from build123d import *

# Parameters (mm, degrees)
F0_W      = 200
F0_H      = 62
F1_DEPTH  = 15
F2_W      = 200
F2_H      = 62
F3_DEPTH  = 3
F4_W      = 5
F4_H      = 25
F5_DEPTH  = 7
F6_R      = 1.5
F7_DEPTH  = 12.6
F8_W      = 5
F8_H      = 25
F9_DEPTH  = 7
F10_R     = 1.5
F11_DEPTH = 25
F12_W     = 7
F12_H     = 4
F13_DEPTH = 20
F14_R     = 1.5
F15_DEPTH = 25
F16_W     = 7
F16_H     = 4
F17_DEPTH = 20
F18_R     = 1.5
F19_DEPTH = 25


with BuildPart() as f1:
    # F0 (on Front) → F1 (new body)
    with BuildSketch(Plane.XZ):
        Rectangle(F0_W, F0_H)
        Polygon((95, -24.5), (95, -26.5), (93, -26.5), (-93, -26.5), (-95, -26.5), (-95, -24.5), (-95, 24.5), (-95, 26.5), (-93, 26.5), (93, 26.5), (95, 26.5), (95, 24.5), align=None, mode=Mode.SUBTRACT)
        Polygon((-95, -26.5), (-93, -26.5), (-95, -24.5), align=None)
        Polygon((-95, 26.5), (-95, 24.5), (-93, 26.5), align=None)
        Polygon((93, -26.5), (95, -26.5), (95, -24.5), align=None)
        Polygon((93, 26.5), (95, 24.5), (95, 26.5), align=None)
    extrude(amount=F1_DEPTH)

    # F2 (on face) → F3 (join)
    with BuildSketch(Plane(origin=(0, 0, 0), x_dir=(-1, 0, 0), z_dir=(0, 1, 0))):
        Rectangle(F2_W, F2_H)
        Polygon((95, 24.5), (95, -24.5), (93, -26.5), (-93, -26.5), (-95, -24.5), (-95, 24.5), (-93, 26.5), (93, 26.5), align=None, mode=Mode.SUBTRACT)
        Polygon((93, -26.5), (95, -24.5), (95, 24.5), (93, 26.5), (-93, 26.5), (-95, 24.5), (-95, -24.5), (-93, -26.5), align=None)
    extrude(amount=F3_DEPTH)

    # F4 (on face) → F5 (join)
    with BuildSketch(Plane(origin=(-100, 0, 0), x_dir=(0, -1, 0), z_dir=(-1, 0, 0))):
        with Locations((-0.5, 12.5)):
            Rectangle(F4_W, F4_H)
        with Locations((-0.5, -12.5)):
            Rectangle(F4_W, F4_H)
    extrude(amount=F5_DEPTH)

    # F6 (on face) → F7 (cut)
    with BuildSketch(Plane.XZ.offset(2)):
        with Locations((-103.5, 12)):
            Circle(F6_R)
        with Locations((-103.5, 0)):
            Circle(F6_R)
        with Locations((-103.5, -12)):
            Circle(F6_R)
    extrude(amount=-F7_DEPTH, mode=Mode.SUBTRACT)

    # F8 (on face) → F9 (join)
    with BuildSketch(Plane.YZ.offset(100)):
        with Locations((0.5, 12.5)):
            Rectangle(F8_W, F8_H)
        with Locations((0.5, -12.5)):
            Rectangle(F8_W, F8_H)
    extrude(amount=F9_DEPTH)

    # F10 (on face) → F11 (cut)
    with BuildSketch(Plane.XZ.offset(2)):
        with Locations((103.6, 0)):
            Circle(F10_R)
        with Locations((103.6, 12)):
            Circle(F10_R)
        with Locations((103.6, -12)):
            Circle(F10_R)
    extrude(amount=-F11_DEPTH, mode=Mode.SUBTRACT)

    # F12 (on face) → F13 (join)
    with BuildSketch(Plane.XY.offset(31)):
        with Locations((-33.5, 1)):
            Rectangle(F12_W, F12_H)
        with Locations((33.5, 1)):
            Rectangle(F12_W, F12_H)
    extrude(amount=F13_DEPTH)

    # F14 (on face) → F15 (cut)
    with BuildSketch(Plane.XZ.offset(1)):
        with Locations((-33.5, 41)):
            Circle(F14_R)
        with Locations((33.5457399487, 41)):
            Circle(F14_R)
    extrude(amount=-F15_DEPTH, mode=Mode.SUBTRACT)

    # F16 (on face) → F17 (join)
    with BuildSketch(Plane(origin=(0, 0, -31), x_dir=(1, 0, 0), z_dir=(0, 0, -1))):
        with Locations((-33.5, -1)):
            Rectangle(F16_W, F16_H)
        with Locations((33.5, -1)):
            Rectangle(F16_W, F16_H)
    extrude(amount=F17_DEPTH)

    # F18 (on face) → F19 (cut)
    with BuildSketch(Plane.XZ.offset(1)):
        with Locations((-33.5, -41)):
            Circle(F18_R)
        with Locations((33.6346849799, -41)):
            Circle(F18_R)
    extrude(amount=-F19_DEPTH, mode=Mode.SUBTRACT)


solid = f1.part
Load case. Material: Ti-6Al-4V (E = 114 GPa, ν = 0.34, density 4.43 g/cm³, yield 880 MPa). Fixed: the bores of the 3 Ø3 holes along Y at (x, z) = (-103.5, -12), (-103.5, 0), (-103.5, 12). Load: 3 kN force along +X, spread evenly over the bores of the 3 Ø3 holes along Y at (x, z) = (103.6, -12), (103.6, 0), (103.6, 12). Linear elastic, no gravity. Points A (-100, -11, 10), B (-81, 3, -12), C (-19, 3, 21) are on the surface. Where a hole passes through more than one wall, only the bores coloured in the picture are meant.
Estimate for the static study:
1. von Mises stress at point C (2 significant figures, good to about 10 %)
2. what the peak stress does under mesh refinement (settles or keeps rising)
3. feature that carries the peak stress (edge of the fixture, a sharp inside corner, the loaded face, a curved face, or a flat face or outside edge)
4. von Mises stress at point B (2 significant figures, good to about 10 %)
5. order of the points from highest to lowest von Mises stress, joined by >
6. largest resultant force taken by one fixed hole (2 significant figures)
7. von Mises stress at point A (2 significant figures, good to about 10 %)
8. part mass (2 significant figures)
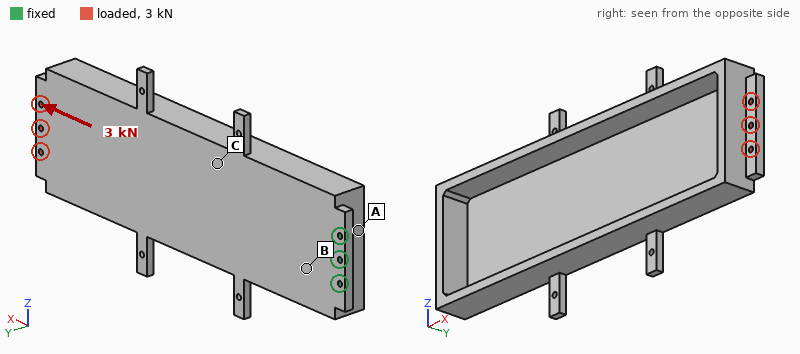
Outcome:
14 MPa
keeps rising
edge of the fixture
19 MPa
B > C > A
1.2 kN
6.3 MPa
340 g
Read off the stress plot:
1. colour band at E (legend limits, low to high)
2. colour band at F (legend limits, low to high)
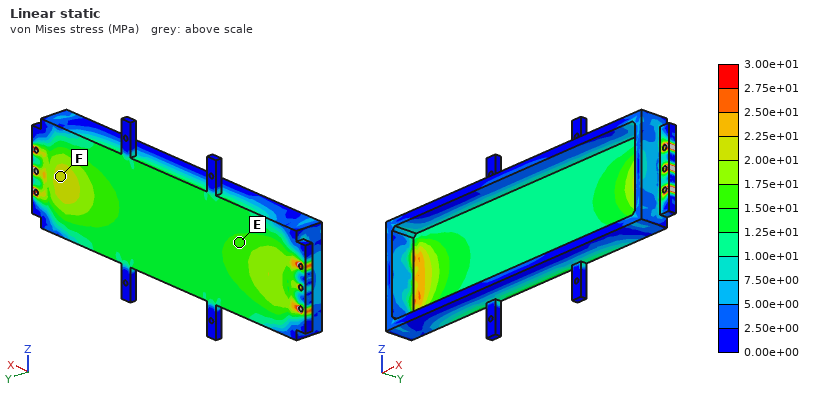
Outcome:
1.50e+01 to 1.75e+01 MPa
2.00e+01 to 2.25e+01 MPa
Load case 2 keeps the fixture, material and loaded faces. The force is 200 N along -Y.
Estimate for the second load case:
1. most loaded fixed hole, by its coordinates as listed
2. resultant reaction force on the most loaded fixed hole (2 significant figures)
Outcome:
(-103.5, 0)
880 N
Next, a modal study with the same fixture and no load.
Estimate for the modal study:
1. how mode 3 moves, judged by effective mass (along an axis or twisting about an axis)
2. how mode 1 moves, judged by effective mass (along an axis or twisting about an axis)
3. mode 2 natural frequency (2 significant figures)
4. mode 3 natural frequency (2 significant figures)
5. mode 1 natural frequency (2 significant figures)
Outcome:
along Z
along Y
400 Hz
660 Hz
140 Hz
